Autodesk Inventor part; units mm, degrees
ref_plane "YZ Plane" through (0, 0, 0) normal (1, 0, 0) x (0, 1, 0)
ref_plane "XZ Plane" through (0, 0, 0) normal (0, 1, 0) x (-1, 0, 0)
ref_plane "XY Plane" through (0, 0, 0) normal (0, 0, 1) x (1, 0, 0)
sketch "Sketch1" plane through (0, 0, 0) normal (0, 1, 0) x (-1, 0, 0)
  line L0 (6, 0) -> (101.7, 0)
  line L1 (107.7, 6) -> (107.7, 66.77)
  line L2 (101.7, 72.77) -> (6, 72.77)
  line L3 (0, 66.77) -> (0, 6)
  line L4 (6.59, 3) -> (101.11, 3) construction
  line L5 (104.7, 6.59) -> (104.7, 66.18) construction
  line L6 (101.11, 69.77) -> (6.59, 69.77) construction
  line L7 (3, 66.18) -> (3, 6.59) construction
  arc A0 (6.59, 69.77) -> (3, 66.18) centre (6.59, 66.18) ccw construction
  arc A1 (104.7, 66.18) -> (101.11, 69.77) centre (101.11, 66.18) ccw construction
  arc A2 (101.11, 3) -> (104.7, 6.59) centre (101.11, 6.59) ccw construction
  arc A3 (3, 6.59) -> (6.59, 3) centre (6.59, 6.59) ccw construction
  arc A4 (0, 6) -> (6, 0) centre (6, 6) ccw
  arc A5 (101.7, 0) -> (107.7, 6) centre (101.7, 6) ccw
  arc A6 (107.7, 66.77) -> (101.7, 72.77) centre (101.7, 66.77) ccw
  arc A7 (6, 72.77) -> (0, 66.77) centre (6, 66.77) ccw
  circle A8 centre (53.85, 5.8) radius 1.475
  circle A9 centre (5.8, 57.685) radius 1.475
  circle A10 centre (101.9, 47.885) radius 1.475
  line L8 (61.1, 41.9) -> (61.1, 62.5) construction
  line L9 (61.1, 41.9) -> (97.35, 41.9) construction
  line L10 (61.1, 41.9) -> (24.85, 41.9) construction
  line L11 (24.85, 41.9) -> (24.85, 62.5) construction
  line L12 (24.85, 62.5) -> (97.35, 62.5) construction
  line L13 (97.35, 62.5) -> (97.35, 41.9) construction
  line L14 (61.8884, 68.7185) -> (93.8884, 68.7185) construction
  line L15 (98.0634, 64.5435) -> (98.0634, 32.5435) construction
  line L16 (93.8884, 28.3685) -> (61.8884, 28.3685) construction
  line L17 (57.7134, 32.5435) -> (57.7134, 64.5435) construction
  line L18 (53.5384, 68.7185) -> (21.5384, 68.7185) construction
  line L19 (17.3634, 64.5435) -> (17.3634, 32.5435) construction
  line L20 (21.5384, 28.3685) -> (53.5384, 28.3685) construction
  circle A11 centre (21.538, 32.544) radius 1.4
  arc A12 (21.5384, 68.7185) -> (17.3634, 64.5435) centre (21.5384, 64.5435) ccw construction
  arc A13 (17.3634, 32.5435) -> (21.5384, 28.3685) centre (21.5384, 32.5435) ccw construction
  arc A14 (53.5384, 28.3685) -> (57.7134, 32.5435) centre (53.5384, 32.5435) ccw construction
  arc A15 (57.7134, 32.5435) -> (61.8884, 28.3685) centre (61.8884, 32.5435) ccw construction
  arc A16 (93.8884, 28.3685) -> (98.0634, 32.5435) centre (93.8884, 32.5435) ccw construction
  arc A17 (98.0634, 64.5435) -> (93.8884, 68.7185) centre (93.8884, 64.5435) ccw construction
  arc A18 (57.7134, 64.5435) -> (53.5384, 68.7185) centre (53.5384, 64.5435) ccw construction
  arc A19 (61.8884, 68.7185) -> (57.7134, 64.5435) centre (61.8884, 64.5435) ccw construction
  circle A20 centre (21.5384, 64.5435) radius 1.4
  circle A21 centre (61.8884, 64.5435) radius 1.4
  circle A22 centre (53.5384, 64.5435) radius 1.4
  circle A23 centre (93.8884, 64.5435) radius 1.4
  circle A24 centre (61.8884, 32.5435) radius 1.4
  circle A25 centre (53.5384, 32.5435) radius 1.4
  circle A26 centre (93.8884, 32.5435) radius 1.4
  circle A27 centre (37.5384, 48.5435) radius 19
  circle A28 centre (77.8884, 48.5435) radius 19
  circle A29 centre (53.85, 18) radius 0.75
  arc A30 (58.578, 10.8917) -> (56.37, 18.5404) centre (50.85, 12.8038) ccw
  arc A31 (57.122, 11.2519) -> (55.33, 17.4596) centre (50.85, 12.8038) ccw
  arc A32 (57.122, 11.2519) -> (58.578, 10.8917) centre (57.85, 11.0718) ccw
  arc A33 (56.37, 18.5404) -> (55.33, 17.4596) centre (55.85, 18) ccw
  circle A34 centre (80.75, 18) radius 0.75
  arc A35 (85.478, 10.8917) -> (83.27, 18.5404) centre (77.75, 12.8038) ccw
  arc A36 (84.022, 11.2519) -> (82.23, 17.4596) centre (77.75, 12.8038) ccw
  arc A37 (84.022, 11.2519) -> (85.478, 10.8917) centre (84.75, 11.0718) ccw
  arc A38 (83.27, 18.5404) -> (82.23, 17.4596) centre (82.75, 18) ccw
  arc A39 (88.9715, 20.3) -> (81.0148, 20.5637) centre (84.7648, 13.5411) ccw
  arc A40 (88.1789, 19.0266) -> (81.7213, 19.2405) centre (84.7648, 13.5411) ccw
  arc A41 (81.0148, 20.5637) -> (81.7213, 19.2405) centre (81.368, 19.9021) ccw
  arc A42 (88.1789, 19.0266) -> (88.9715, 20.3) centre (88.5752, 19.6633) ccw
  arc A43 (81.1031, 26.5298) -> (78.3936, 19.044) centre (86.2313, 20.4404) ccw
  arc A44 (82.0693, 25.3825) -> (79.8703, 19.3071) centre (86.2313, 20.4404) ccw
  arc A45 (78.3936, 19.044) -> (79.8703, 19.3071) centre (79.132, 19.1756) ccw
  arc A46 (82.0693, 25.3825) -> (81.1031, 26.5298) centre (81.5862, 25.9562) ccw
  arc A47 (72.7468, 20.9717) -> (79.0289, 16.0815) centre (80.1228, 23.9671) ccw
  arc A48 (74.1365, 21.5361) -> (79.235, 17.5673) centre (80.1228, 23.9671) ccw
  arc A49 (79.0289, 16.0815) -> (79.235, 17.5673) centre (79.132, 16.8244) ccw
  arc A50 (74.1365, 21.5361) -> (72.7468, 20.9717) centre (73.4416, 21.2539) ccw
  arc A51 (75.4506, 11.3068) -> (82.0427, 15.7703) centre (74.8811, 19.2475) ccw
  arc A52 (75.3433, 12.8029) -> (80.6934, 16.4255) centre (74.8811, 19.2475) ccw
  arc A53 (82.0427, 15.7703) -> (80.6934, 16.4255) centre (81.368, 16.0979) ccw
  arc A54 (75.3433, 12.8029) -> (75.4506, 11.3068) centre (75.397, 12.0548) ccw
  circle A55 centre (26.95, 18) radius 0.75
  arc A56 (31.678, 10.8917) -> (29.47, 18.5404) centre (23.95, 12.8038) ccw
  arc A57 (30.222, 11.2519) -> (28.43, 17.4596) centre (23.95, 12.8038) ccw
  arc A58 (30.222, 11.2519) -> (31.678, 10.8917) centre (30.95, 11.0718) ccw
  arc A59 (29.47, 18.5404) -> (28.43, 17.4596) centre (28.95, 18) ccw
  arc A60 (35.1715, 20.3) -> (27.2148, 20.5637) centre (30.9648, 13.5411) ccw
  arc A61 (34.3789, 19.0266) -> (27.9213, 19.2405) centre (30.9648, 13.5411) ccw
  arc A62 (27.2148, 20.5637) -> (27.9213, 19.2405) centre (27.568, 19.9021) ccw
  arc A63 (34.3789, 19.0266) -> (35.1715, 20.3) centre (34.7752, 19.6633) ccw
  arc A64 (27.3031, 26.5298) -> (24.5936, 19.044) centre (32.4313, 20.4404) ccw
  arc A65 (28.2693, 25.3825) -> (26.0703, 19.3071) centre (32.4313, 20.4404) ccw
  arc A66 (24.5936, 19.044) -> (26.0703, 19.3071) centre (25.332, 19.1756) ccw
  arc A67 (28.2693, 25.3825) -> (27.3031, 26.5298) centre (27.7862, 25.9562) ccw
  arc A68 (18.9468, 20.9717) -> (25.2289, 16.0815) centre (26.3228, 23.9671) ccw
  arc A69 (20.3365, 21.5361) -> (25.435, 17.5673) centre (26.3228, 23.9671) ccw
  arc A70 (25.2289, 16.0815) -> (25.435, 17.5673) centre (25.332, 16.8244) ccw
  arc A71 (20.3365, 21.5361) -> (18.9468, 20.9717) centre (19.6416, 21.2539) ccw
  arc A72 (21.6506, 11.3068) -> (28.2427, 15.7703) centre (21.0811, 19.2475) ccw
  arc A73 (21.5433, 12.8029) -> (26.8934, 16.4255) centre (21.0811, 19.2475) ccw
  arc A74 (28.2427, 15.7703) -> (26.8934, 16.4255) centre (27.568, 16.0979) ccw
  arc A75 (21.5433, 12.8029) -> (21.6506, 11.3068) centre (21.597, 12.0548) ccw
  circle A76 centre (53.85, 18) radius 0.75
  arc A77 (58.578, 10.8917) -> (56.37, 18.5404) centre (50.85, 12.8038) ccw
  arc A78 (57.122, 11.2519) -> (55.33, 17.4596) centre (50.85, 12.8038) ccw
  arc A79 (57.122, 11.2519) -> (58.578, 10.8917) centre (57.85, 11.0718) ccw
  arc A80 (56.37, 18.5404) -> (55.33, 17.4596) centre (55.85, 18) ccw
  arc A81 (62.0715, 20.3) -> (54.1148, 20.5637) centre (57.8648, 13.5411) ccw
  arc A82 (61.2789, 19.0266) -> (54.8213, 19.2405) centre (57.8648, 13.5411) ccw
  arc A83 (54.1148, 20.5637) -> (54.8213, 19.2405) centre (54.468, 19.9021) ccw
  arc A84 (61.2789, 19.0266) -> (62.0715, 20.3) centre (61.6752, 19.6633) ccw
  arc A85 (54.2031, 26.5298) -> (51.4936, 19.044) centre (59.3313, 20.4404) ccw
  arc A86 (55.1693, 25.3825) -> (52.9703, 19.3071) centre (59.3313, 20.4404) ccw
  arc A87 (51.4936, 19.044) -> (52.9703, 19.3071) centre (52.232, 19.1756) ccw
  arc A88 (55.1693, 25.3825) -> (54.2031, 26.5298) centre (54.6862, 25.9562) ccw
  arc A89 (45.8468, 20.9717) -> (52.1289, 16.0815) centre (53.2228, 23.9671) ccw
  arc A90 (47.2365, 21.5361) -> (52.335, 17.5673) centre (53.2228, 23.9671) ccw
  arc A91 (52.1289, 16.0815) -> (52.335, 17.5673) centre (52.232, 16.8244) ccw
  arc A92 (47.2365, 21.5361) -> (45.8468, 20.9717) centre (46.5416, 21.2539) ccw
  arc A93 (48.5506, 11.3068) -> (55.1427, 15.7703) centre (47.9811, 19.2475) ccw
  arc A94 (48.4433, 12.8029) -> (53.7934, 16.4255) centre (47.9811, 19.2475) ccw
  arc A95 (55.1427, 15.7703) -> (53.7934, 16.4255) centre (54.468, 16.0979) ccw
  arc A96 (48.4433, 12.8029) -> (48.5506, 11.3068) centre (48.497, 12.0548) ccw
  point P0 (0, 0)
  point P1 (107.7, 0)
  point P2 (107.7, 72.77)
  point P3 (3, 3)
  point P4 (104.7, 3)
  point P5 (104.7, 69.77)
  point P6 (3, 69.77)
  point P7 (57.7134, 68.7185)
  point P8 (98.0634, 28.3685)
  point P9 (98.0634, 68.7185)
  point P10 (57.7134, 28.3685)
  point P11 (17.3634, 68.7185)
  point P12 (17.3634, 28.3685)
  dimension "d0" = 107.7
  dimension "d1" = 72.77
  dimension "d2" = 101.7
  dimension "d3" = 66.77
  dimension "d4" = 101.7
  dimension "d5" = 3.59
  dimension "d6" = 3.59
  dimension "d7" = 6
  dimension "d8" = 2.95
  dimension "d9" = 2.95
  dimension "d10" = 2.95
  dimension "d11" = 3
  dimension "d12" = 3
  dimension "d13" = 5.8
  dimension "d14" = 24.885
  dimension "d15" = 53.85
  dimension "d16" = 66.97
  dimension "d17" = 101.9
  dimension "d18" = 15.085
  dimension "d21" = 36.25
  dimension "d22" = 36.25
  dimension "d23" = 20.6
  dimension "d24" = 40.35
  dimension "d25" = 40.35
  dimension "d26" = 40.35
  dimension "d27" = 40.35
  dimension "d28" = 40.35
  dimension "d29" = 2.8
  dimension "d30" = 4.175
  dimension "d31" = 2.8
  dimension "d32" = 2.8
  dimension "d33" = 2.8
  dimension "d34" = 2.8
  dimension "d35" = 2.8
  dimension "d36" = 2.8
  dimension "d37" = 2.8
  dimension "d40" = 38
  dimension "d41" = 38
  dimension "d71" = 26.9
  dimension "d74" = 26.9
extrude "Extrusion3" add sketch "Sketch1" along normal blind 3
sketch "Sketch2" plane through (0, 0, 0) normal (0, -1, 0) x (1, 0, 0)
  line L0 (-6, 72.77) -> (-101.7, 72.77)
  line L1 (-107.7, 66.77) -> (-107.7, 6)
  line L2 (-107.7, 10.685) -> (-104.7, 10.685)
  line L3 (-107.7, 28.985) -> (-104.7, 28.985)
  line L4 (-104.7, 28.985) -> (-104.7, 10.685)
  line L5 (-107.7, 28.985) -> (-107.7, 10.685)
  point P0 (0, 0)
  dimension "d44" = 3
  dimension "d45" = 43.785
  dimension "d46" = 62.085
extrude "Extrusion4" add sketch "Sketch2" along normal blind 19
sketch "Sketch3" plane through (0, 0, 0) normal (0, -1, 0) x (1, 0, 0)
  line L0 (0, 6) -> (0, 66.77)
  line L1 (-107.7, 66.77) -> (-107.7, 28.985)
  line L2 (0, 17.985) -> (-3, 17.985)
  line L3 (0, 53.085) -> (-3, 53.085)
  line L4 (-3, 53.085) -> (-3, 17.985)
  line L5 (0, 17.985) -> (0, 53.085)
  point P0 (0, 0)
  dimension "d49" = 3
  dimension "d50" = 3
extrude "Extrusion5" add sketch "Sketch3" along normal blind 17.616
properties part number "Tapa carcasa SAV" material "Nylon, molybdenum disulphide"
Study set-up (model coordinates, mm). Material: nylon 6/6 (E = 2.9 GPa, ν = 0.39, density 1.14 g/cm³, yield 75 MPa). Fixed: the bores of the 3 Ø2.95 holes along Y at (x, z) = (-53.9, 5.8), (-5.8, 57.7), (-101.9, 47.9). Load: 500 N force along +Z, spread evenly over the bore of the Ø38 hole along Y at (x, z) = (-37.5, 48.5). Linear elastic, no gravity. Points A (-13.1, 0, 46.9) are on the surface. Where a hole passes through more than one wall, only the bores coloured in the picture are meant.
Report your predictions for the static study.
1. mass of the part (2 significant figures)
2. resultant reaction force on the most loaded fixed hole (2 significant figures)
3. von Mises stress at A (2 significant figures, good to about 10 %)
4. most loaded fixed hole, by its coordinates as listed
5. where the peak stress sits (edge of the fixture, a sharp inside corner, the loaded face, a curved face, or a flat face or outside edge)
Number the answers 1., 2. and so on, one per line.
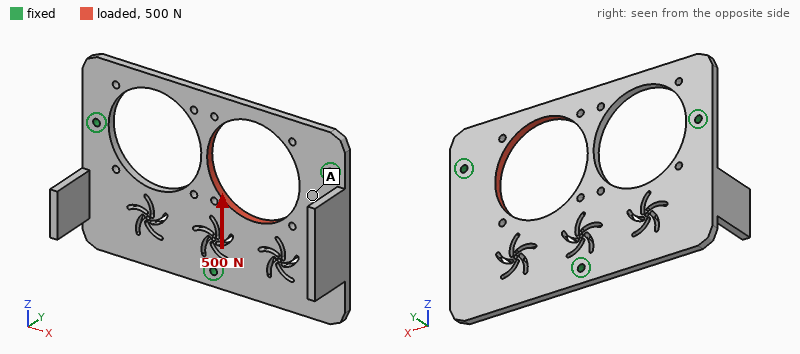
1. 21 g
2. 260 N
3. 4.5 MPa
4. (-5.8, 57.7)
5. a curved face
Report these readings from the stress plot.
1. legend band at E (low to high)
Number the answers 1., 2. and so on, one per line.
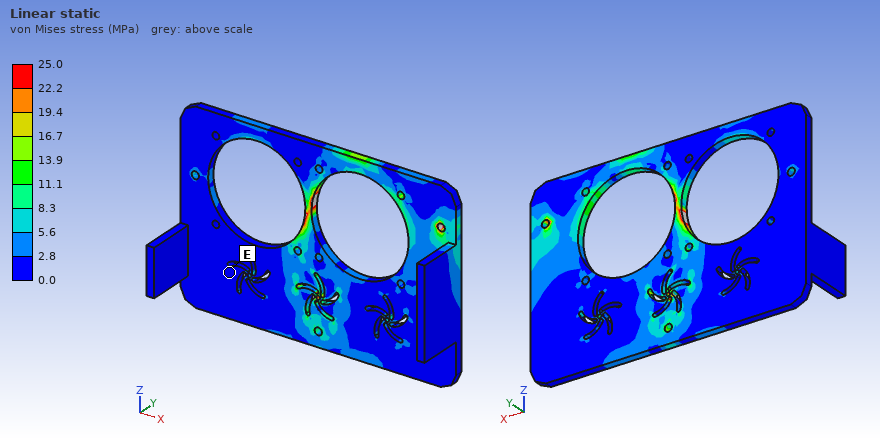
1. 0.0 to 2.8 MPa
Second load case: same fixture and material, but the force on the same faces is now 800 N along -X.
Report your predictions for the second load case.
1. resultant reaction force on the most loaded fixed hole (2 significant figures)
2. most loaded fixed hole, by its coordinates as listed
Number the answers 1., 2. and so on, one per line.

1. 470 N
2. (-5.8, 57.7)
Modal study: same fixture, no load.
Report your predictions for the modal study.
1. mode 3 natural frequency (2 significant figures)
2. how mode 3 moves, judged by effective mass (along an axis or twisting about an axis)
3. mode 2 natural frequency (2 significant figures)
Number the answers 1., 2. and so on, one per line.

1. 500 Hz
2. along Y
3. 400 Hz
